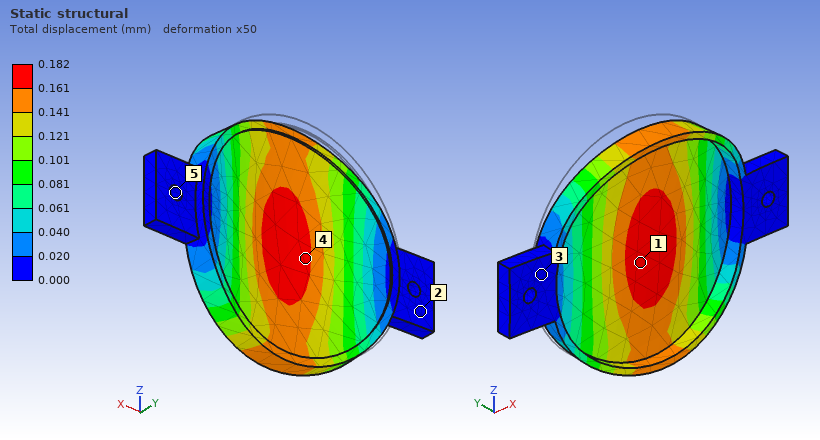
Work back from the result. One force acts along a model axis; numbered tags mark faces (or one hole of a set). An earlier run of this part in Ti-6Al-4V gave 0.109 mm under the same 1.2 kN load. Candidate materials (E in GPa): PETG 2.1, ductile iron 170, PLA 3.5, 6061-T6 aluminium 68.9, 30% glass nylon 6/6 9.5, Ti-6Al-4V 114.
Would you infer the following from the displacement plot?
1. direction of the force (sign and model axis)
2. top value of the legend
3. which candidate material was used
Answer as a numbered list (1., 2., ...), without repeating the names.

1. -Y
2. 0.182 mm
3. 6061-T6 aluminium
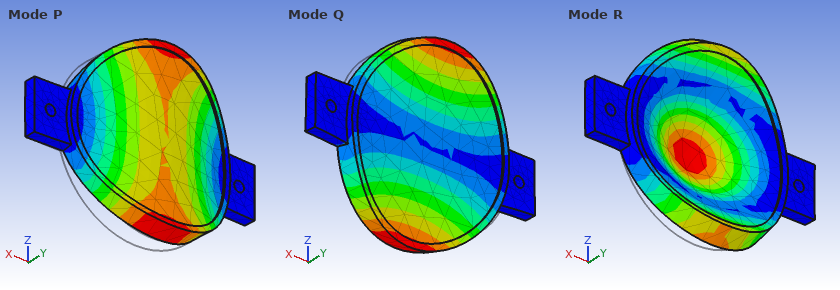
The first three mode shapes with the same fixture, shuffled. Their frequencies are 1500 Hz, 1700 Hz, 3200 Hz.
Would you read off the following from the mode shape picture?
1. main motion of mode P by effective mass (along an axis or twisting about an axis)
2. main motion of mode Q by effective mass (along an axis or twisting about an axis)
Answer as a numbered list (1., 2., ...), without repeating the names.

1. along Y
2. twisting about X
